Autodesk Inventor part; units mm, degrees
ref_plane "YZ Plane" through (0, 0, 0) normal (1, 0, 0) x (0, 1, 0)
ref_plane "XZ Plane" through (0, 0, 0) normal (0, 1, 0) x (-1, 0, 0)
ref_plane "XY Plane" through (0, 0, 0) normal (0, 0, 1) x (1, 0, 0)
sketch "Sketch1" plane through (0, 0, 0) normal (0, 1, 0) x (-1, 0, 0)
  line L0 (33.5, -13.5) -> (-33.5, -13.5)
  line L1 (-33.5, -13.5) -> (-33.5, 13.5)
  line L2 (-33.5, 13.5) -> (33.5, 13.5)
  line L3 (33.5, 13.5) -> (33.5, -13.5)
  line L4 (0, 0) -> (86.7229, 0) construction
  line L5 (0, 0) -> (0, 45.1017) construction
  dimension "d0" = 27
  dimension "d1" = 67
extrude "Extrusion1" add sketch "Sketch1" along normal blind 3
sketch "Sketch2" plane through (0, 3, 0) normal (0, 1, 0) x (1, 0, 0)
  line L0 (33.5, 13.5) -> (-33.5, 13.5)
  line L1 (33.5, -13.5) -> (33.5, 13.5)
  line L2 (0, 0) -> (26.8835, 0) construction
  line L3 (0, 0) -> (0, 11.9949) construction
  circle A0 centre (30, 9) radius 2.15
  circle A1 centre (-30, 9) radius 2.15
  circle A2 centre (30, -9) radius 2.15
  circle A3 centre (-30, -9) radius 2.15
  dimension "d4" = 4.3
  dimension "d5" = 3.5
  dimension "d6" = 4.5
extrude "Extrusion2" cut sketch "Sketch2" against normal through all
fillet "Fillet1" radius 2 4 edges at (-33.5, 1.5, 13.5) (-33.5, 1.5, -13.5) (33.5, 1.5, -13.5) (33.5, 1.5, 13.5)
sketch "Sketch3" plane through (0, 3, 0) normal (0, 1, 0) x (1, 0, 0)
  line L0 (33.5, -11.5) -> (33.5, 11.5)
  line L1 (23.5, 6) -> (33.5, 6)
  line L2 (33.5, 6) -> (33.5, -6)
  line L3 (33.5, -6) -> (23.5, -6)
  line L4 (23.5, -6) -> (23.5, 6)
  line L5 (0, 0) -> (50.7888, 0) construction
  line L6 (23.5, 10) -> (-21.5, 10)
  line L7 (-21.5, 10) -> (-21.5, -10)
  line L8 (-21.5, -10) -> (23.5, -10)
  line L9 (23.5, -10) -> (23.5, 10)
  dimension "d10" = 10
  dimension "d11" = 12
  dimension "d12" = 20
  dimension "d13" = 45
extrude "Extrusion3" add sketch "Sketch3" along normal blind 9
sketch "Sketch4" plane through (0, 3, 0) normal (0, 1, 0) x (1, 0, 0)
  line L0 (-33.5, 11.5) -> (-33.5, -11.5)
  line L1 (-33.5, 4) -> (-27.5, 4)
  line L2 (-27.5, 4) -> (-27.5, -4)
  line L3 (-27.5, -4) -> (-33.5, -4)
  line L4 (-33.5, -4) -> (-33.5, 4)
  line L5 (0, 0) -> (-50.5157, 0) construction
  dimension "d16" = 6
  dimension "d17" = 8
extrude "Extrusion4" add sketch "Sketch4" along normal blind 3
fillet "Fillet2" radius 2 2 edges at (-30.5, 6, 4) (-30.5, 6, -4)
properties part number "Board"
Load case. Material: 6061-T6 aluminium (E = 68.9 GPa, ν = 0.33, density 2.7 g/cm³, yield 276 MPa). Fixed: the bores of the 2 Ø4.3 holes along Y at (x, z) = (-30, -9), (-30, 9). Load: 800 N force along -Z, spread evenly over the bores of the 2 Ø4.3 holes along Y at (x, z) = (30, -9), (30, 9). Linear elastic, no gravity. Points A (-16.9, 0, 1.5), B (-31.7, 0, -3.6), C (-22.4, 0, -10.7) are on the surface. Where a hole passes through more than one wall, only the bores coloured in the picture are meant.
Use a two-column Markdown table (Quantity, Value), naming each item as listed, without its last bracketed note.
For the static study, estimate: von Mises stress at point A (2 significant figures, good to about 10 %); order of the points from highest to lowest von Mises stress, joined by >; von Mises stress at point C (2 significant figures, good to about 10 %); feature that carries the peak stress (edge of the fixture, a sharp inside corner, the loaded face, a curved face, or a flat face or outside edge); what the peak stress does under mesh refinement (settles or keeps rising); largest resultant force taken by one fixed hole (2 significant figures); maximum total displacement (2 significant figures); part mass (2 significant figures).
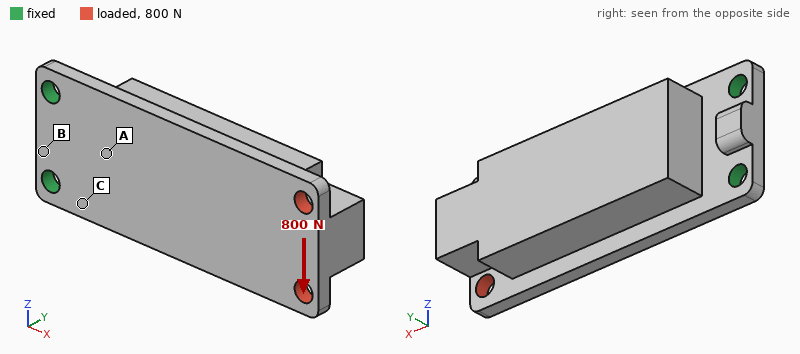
| Quantity | Value |
|---|---|
| von Mises stress at point A | 38 MPa |
| order of the points from highest to lowest von Mises stress, joined by > | C > A > B |
| von Mises stress at point C | 81 MPa |
| feature that carries the peak stress | edge of the fixture |
| what the peak stress does under mesh refinement | keeps rising |
| largest resultant force taken by one fixed hole | 2.4 kN |
| maximum total displacement | 0.17 mm |
| part mass | 39 g |
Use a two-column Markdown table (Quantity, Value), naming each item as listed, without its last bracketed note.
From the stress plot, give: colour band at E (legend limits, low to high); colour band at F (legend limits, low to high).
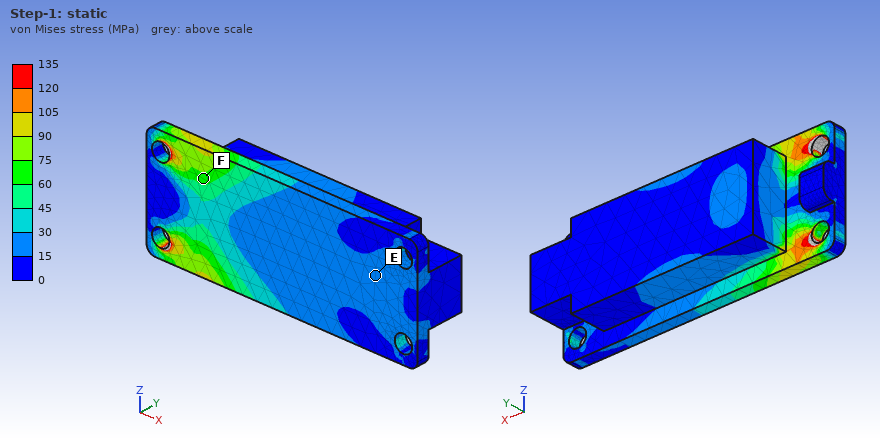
| Quantity | Value |
|---|---|
| colour band at E | 15 to 30 MPa |
| colour band at F | 60 to 75 MPa |
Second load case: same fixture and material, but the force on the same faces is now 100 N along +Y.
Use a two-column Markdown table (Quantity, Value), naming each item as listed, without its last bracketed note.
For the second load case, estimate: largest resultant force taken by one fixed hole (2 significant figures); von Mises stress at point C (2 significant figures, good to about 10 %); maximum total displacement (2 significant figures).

| Quantity | Value |
|---|---|
| largest resultant force taken by one fixed hole | 66 N |
| von Mises stress at point C | 110 MPa |
| maximum total displacement | 0.70 mm |
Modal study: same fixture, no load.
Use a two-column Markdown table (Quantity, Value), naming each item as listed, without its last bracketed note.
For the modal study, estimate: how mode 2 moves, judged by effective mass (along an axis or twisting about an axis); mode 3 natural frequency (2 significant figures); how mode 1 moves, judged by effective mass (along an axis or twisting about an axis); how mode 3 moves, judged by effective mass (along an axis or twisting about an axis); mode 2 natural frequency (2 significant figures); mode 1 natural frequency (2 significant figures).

| Quantity | Value |
|---|---|
| how mode 2 moves, judged by effective mass | along Z |
| mode 3 natural frequency | 5500 Hz |
| how mode 1 moves, judged by effective mass | along Y |
| how mode 3 moves, judged by effective mass | twisting about X |
| mode 2 natural frequency | 3300 Hz |
| mode 1 natural frequency | 540 Hz |
